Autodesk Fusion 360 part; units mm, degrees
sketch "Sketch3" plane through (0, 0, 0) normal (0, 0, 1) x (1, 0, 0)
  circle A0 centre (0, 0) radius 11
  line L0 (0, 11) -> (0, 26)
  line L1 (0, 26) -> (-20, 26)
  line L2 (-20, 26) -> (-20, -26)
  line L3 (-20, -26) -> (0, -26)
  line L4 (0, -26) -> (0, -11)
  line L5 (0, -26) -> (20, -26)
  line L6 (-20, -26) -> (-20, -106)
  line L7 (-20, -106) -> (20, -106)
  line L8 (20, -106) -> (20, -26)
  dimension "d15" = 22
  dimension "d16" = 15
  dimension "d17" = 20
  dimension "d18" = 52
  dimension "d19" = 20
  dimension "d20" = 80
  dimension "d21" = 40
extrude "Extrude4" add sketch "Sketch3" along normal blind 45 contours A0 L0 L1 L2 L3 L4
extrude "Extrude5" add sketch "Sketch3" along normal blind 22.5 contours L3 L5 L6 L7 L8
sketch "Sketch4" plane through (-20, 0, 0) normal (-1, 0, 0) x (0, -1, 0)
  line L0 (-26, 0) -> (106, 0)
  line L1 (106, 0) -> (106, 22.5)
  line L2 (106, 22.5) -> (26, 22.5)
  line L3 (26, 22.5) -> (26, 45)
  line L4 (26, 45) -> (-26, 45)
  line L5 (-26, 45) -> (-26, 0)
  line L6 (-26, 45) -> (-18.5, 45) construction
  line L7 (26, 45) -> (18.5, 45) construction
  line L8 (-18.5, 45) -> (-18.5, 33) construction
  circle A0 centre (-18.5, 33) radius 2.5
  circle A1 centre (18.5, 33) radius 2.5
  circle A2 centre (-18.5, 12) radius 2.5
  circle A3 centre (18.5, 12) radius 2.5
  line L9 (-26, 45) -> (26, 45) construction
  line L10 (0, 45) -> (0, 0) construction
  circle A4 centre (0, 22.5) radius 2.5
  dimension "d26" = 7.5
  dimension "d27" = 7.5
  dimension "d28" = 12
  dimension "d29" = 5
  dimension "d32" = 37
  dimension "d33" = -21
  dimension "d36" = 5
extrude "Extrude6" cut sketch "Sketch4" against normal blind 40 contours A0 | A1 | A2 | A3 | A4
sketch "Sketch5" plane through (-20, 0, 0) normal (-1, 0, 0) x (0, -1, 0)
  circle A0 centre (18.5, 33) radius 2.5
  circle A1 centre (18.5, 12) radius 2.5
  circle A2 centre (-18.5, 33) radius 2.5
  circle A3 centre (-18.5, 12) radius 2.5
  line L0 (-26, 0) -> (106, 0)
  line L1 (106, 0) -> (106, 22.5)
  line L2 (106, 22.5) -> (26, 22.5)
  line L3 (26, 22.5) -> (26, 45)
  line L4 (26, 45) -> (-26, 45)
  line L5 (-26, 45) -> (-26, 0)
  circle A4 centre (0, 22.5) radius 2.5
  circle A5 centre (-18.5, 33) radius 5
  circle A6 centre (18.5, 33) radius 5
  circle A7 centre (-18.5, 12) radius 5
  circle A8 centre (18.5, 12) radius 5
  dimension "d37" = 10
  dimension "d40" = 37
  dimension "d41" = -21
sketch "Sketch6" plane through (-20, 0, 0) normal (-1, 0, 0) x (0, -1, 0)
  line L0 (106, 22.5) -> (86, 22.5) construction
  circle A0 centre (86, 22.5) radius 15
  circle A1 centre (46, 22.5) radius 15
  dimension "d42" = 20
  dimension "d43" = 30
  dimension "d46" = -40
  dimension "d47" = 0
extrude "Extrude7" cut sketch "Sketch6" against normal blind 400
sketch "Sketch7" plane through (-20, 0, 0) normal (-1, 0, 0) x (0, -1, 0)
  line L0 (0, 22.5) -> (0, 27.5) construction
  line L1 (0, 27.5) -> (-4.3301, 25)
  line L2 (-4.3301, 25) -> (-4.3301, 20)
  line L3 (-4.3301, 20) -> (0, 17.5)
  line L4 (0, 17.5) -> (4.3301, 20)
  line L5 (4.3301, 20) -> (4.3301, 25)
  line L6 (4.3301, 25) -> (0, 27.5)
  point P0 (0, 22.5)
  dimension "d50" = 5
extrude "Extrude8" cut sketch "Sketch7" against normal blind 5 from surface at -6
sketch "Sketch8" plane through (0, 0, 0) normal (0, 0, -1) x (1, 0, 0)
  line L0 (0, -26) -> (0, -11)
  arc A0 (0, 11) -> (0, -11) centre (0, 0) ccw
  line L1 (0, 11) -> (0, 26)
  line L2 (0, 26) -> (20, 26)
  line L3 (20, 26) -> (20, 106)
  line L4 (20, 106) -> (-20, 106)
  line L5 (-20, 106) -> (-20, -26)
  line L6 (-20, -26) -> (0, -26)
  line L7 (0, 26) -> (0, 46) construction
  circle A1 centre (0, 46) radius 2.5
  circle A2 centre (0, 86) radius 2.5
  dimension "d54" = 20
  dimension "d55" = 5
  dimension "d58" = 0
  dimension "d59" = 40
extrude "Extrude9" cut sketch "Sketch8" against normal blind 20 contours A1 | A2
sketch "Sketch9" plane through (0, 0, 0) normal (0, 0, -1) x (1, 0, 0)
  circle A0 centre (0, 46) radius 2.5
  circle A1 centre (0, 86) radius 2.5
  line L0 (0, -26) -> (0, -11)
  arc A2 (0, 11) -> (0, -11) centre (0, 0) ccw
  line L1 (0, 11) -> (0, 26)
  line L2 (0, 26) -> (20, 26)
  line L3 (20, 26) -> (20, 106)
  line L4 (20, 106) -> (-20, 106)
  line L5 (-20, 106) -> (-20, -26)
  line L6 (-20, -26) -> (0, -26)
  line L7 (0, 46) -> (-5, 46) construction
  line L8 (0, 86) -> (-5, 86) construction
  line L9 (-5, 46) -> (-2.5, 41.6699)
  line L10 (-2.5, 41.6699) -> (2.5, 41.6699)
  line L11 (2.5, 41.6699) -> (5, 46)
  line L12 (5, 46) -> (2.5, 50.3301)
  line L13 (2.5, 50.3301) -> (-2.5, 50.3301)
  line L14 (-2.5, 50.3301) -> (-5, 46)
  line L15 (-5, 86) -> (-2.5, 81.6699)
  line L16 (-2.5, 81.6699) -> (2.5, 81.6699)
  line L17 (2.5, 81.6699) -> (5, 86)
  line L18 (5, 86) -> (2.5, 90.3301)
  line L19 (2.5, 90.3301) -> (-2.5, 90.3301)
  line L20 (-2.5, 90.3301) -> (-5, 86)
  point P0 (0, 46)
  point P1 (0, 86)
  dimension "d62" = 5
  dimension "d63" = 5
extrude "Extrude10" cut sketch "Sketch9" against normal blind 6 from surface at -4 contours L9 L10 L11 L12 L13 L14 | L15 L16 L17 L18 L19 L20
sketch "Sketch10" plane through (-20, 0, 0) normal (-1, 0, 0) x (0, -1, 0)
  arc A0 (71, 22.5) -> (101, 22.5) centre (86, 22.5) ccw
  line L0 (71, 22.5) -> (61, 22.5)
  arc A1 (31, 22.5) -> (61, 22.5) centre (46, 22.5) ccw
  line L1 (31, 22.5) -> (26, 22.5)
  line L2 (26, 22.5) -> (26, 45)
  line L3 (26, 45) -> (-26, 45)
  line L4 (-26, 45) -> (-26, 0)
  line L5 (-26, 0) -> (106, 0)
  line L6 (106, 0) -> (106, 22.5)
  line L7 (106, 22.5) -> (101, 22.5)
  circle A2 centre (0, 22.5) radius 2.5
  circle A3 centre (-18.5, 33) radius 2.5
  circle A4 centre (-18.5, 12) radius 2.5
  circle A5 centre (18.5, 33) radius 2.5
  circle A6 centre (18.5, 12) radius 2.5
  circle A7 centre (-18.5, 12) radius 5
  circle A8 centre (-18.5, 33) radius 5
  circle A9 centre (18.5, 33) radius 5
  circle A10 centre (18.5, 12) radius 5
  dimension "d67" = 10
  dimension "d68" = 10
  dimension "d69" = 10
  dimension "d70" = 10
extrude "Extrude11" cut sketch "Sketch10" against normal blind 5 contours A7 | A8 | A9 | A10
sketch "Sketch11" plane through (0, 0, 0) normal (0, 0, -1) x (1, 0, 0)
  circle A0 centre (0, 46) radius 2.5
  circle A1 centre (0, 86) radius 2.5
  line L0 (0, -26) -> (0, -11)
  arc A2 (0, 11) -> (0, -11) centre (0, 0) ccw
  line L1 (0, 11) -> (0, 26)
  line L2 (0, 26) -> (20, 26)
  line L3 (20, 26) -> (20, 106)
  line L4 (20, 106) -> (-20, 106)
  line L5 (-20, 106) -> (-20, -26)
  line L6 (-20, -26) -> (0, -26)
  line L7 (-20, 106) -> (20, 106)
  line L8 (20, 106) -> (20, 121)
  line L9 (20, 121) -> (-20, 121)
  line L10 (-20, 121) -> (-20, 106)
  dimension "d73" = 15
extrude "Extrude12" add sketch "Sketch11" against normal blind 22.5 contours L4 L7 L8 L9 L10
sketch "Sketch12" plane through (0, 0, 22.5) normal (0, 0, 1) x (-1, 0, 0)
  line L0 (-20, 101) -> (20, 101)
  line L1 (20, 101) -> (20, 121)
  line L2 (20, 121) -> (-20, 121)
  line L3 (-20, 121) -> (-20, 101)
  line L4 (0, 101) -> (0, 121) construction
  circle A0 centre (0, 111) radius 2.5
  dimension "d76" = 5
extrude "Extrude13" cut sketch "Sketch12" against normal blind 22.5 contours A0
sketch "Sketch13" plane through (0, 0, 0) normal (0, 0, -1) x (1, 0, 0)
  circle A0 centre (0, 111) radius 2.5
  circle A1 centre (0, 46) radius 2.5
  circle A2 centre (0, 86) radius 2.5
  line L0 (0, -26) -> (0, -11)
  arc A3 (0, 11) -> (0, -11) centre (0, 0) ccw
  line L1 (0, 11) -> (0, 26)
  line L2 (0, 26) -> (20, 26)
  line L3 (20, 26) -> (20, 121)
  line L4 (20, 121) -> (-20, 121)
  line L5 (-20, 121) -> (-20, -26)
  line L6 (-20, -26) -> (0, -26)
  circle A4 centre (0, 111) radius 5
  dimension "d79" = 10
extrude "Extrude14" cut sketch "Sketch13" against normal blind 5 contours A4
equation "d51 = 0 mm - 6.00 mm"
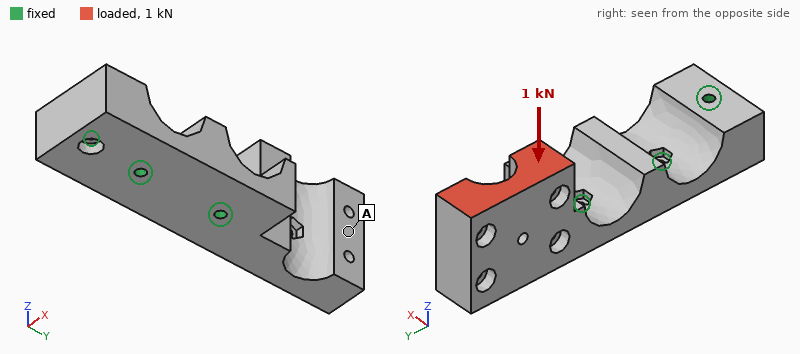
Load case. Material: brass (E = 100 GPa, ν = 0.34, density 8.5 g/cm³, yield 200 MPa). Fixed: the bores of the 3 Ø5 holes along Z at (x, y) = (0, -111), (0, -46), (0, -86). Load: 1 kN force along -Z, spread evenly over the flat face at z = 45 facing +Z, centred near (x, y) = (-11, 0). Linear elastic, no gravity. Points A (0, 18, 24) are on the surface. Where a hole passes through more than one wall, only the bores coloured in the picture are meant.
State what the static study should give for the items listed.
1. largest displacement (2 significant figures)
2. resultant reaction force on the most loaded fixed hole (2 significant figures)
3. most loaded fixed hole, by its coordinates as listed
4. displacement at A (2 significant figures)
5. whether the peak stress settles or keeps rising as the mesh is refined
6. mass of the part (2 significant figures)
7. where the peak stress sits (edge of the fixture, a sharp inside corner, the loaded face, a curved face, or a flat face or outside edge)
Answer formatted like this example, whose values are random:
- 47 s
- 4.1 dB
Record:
- 0.41 mm
- 2.6 kN
- (0, -46)
- 0.31 mm
- keeps rising
- 770 g
- edge of the fixture
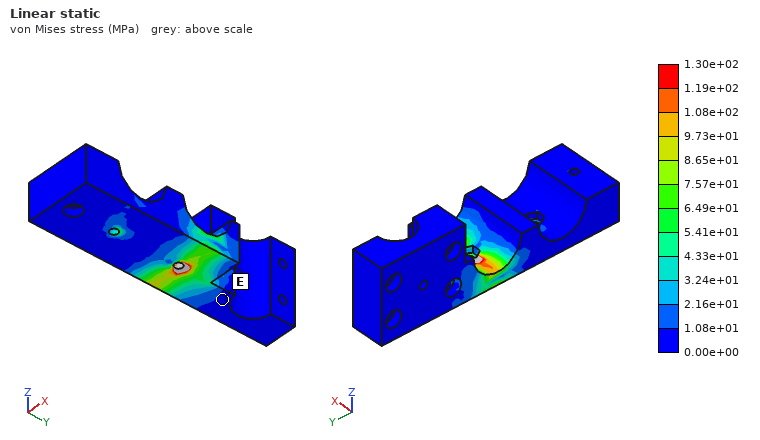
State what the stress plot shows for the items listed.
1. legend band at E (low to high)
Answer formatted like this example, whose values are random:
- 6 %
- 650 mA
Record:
- 0.00e+00 to 1.08e+01 MPa
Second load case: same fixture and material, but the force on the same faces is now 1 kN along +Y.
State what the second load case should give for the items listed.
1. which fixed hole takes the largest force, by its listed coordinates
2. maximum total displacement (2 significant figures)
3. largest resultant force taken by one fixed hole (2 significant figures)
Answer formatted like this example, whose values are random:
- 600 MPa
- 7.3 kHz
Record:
- (0, -86)
- 0.39 mm
- 1.7 kN
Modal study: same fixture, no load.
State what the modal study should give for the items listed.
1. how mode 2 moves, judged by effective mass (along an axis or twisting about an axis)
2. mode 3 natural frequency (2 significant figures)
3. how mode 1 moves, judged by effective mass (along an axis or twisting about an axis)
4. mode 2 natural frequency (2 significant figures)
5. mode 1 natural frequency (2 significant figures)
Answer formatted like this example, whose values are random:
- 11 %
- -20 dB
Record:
- along X
- 2000 Hz
- along Z
- 950 Hz
- 520 Hz
